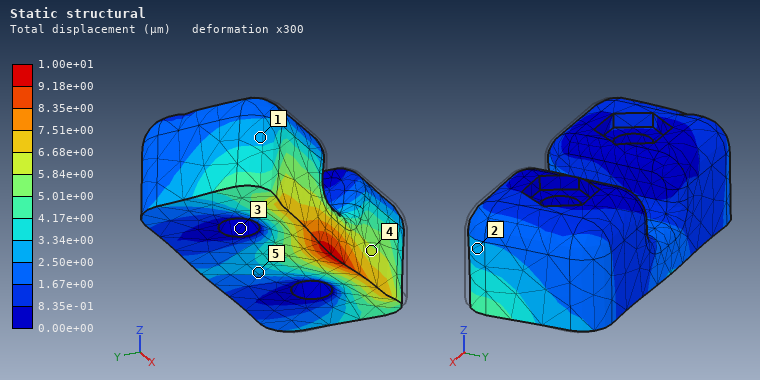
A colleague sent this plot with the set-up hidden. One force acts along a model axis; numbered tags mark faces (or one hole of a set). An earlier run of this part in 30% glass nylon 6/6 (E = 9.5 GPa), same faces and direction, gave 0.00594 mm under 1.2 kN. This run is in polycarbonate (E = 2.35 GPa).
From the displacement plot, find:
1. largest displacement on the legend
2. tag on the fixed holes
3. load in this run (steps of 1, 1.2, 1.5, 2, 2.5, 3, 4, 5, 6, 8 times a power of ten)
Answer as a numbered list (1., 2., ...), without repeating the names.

1. 1.00e+01 µm
2. 3
3. 500 N
